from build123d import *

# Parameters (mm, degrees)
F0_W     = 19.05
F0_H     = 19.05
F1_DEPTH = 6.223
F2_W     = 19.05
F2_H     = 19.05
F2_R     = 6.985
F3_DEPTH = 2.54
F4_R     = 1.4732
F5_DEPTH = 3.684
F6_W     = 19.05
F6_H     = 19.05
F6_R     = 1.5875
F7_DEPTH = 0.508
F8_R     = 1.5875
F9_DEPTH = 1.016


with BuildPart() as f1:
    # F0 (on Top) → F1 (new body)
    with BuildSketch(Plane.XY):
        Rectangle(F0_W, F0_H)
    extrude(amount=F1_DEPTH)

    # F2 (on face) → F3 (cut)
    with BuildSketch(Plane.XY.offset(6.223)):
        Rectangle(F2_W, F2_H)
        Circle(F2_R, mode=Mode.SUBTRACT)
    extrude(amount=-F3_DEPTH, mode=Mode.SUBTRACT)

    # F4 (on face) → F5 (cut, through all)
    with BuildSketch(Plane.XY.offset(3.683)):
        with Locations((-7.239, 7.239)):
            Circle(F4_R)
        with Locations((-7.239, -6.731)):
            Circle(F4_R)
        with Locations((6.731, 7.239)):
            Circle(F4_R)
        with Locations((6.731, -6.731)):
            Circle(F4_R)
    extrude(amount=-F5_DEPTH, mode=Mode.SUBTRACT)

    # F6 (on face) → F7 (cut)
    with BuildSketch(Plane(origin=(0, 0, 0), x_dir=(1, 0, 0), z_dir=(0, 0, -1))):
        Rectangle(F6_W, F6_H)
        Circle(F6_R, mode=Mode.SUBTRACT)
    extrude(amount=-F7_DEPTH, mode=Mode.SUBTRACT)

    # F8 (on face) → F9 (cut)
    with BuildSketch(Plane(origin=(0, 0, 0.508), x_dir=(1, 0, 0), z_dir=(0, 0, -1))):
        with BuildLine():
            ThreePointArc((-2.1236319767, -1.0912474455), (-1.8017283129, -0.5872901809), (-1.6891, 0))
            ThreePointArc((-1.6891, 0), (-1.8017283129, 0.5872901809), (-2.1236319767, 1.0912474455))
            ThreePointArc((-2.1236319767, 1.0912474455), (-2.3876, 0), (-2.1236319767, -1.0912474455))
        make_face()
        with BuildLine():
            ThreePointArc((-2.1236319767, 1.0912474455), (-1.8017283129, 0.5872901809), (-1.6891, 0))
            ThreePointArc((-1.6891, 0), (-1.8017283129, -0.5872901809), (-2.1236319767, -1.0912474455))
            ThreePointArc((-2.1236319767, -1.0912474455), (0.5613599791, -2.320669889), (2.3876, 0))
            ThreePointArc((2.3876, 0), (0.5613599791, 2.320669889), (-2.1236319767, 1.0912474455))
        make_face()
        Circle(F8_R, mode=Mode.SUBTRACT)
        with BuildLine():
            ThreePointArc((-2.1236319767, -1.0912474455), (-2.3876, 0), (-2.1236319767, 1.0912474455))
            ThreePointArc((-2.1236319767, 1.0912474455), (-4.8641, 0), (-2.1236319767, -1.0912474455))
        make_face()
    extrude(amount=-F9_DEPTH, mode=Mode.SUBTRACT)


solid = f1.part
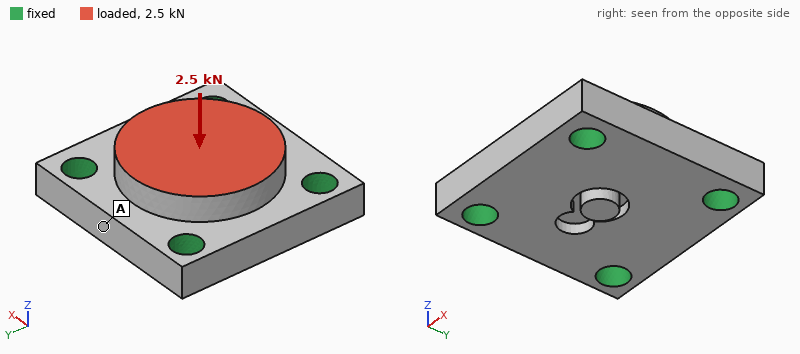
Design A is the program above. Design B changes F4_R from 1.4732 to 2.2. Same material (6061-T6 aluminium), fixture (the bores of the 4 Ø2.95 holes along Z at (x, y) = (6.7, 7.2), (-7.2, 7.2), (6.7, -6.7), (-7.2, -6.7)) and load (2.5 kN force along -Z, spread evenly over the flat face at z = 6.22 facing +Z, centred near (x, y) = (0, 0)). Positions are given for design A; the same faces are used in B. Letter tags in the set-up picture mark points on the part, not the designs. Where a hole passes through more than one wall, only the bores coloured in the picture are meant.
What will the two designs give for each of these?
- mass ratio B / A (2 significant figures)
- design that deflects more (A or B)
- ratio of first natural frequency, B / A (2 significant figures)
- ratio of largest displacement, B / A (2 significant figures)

0.93
A
1.2
0.70
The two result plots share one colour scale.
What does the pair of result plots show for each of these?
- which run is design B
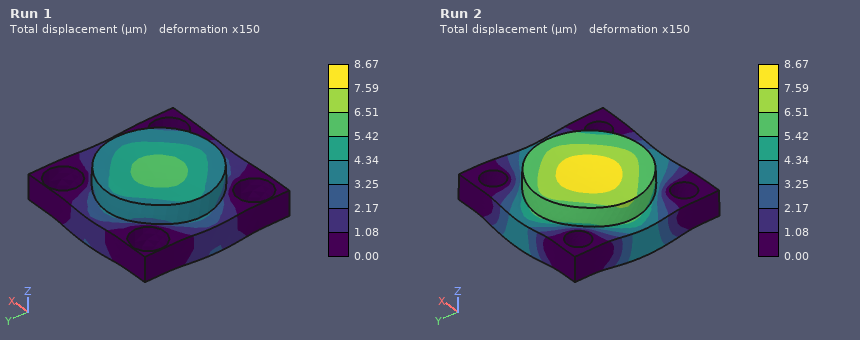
Run 1
